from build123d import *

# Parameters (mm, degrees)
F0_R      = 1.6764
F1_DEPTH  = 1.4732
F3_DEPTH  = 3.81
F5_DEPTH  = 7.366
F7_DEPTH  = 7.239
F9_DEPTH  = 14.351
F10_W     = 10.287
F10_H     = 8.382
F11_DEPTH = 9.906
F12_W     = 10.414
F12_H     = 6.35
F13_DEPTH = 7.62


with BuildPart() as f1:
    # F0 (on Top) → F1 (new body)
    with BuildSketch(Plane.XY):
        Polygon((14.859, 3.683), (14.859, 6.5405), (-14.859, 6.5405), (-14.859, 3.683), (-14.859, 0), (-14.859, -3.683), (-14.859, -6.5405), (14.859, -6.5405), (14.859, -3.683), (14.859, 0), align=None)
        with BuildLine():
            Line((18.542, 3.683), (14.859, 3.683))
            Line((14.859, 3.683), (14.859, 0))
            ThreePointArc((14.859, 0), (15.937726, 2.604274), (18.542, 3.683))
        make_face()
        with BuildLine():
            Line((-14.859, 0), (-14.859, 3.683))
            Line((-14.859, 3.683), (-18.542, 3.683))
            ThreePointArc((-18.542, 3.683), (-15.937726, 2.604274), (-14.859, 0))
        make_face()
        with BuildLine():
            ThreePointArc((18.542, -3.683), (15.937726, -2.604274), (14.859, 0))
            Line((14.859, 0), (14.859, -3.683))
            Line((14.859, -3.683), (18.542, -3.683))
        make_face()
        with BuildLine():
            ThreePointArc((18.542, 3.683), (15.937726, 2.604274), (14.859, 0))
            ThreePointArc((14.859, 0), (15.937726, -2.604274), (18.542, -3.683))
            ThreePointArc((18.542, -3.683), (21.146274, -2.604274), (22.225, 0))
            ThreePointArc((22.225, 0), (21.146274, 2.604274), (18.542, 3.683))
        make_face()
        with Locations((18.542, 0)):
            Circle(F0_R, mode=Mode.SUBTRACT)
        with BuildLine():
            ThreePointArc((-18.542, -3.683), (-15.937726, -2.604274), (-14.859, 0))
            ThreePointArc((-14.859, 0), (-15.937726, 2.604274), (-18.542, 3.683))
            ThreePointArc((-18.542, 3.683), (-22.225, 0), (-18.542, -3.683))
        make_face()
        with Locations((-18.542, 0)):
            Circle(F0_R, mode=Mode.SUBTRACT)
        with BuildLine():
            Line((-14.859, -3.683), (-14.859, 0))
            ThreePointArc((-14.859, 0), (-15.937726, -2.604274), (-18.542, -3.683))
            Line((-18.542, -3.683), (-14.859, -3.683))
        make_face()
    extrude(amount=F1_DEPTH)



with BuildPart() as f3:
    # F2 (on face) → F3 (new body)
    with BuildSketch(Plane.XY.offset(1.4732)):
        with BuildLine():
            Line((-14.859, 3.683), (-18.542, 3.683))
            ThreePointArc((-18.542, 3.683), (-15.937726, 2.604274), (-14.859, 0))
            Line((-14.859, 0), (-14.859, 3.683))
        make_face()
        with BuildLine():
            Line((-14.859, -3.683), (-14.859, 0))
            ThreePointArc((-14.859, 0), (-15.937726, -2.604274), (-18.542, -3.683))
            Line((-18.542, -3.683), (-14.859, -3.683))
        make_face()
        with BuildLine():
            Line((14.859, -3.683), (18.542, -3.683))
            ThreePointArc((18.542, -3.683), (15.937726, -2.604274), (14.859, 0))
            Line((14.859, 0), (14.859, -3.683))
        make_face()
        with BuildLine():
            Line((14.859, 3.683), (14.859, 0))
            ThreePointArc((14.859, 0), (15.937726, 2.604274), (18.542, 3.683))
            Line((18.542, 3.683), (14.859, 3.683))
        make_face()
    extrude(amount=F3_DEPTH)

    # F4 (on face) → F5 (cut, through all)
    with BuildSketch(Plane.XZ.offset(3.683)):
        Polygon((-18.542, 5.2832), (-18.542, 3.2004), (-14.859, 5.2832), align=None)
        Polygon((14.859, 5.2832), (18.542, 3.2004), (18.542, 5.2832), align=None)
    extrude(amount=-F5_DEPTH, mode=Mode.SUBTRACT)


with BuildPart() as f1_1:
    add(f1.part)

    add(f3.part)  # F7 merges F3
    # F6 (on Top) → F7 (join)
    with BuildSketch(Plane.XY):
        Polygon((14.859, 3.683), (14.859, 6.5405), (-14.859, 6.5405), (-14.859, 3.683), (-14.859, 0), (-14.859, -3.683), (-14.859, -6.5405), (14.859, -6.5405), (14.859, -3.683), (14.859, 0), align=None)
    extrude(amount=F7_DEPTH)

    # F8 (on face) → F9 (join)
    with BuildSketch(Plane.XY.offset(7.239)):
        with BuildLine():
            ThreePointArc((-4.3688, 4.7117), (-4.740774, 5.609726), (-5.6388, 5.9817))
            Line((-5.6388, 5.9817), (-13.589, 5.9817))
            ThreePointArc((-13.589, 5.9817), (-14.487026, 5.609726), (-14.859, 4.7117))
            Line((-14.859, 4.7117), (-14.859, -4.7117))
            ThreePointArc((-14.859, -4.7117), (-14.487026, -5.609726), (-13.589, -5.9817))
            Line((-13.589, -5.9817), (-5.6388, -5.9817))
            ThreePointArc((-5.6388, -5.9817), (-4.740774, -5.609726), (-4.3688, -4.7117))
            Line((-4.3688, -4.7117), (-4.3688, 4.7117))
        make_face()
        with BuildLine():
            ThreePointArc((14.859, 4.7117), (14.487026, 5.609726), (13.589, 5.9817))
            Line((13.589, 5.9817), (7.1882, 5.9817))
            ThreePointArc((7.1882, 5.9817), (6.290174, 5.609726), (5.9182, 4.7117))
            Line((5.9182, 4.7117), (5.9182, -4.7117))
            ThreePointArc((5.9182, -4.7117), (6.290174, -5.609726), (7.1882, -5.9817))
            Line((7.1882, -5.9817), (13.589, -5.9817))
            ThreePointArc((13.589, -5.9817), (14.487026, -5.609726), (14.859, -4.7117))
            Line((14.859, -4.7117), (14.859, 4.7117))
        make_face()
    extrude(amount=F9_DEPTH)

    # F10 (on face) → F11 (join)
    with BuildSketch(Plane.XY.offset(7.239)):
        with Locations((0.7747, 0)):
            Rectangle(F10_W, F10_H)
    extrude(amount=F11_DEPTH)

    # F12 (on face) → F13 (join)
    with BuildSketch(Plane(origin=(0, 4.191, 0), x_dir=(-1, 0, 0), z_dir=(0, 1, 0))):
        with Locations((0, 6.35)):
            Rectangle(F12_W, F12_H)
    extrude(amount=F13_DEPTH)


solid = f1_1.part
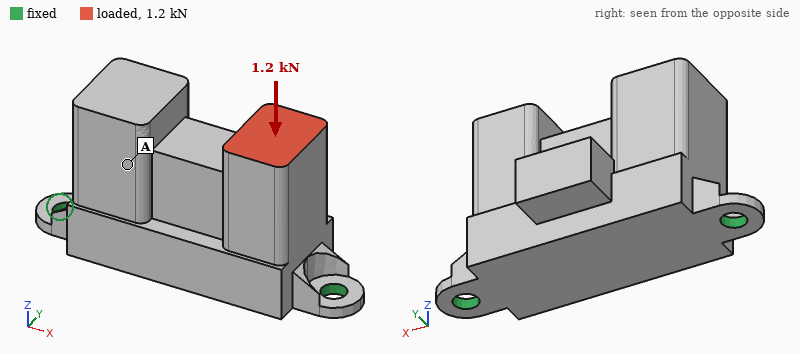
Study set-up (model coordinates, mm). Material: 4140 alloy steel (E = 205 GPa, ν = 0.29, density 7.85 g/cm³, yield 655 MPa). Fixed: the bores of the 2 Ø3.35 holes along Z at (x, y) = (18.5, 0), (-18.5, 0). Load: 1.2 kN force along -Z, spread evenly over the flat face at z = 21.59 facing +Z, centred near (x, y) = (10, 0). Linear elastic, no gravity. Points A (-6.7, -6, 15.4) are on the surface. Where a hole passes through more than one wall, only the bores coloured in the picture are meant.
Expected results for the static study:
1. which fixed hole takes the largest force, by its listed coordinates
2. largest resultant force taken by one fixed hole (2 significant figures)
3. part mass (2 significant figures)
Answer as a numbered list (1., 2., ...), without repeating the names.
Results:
1. (18.5, 0)
2. 1.0 kN
3. 59 g
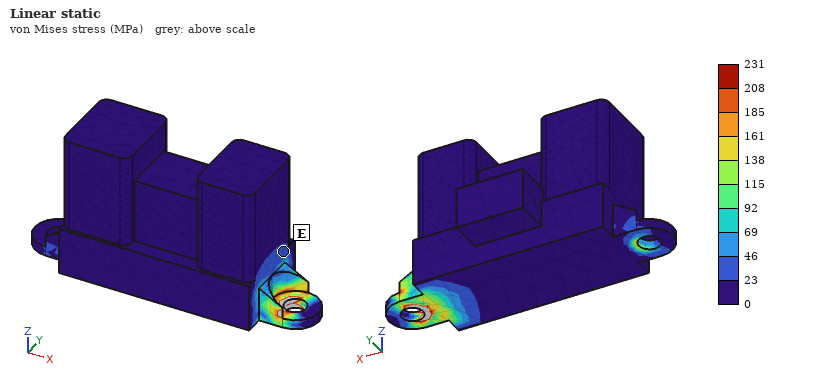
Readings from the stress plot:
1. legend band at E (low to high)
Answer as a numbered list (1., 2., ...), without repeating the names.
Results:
1. 23 to 46 MPa
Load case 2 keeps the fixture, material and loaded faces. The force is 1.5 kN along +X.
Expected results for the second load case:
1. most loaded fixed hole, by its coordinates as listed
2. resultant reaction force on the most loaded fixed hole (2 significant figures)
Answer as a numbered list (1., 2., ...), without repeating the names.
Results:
1. (-18.5, 0)
2. 1.3 kN
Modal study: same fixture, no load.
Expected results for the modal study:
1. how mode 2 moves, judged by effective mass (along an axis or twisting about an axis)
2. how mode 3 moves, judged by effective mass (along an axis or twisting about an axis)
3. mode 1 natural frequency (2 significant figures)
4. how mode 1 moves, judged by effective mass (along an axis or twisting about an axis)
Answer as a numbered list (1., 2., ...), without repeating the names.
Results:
1. along Z
2. along X
3. 2100 Hz
4. along Y
